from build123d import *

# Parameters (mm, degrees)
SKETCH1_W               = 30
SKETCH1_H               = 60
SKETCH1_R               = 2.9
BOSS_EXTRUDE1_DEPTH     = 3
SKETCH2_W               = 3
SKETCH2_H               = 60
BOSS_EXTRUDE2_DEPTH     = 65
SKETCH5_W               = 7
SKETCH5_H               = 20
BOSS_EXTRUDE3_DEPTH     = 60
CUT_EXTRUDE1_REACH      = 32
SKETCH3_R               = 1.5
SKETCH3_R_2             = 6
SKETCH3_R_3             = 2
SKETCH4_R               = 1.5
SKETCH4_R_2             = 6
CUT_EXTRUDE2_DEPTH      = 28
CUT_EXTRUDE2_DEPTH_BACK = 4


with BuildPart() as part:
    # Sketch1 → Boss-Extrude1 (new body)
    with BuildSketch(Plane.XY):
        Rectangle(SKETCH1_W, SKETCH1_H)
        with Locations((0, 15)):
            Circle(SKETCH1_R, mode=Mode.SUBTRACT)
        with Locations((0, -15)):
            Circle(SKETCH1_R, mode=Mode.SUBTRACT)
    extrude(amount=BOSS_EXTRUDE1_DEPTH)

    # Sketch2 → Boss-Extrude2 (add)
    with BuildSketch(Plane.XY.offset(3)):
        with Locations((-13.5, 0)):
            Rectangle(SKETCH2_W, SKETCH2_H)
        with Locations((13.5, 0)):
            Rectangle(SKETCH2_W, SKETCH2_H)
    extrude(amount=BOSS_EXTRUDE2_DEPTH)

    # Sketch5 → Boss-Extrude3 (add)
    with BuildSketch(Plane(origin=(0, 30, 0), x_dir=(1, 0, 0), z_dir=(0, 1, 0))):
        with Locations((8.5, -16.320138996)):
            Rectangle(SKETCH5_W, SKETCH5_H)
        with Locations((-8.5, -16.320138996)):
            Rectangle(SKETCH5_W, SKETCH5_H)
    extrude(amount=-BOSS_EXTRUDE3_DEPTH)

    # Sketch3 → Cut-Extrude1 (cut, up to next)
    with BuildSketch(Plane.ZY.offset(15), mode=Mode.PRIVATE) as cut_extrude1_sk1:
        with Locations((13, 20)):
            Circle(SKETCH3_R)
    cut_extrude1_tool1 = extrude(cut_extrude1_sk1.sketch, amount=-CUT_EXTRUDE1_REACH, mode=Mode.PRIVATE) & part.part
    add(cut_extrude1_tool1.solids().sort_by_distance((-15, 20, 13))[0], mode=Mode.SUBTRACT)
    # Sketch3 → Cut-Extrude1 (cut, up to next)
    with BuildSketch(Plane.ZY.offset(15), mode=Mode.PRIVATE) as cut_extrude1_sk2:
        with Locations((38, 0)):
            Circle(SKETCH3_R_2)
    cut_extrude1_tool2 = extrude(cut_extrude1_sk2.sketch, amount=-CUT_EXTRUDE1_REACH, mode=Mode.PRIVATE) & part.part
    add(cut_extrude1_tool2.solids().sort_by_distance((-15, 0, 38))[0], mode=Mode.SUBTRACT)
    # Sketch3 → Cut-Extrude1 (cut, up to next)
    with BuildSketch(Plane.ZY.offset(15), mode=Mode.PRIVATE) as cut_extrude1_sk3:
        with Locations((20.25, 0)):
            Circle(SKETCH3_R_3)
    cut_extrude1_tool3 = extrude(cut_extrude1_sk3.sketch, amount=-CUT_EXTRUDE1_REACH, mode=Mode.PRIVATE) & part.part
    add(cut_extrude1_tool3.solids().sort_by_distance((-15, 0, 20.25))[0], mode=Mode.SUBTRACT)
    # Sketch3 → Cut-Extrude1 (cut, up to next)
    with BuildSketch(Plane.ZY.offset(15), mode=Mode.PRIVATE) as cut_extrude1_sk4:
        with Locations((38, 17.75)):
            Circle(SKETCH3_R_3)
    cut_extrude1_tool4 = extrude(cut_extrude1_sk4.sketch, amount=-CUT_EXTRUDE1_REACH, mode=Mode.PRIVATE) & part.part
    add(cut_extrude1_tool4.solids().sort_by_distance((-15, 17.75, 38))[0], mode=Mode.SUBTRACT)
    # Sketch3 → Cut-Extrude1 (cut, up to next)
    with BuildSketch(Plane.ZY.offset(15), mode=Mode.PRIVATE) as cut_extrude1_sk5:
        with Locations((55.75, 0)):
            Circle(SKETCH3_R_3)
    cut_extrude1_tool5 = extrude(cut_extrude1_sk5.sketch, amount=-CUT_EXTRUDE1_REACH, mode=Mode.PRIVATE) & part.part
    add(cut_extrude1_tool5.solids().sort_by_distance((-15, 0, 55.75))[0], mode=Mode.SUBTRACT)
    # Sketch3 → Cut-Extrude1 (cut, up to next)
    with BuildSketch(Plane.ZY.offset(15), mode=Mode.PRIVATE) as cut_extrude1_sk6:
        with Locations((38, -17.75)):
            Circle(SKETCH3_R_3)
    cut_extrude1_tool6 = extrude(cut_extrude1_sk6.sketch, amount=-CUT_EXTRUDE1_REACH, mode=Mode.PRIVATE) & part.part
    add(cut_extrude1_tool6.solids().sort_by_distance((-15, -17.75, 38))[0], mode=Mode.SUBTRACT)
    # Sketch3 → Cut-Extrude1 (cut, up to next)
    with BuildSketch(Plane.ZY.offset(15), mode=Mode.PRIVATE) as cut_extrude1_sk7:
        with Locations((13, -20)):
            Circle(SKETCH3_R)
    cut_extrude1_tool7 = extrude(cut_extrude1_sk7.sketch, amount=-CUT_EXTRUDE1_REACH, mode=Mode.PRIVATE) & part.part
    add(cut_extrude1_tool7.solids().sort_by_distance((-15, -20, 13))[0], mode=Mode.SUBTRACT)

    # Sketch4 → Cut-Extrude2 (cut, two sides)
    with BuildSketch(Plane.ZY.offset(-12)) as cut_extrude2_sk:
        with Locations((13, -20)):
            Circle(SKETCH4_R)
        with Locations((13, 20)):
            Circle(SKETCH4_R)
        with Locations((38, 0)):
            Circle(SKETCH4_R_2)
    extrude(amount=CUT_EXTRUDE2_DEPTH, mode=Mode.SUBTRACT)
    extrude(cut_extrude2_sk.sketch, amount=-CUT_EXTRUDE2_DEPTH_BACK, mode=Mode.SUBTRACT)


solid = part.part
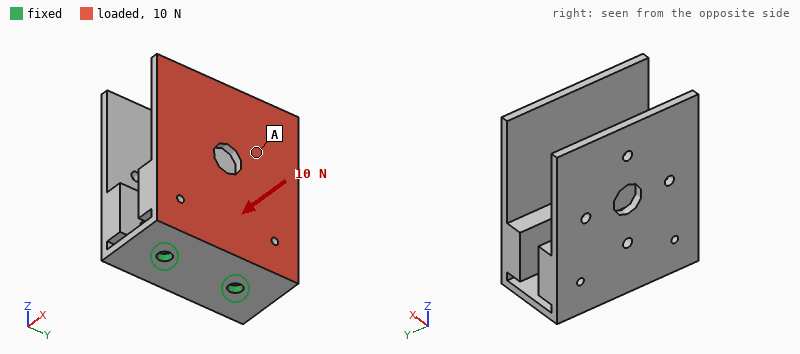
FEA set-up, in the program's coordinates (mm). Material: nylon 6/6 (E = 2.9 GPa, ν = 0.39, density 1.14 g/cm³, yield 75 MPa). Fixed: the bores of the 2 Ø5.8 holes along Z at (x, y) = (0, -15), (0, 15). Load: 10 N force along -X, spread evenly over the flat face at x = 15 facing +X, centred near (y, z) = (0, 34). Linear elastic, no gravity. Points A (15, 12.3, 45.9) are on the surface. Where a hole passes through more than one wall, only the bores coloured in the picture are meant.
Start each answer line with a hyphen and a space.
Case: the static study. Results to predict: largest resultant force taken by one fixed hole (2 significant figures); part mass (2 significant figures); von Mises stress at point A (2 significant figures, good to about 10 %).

- 5.1 N
- 50 g
- 0.43 MPa
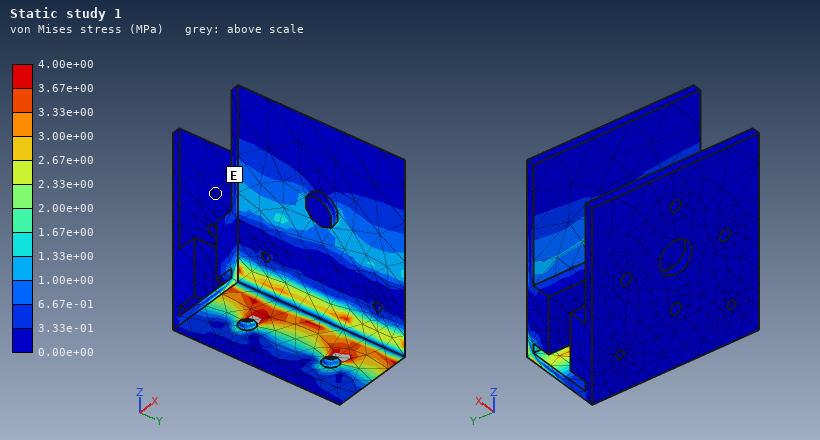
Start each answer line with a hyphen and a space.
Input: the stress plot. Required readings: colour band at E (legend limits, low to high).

- 0.00e+00 to 3.33e-01 MPa
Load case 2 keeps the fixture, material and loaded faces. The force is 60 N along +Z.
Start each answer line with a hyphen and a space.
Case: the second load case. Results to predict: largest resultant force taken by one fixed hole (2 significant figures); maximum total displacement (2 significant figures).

- 30 N
- 1.1 mm
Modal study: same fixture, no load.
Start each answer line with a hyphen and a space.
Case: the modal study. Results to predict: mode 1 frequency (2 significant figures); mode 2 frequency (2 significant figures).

- 160 Hz
- 160 Hz
